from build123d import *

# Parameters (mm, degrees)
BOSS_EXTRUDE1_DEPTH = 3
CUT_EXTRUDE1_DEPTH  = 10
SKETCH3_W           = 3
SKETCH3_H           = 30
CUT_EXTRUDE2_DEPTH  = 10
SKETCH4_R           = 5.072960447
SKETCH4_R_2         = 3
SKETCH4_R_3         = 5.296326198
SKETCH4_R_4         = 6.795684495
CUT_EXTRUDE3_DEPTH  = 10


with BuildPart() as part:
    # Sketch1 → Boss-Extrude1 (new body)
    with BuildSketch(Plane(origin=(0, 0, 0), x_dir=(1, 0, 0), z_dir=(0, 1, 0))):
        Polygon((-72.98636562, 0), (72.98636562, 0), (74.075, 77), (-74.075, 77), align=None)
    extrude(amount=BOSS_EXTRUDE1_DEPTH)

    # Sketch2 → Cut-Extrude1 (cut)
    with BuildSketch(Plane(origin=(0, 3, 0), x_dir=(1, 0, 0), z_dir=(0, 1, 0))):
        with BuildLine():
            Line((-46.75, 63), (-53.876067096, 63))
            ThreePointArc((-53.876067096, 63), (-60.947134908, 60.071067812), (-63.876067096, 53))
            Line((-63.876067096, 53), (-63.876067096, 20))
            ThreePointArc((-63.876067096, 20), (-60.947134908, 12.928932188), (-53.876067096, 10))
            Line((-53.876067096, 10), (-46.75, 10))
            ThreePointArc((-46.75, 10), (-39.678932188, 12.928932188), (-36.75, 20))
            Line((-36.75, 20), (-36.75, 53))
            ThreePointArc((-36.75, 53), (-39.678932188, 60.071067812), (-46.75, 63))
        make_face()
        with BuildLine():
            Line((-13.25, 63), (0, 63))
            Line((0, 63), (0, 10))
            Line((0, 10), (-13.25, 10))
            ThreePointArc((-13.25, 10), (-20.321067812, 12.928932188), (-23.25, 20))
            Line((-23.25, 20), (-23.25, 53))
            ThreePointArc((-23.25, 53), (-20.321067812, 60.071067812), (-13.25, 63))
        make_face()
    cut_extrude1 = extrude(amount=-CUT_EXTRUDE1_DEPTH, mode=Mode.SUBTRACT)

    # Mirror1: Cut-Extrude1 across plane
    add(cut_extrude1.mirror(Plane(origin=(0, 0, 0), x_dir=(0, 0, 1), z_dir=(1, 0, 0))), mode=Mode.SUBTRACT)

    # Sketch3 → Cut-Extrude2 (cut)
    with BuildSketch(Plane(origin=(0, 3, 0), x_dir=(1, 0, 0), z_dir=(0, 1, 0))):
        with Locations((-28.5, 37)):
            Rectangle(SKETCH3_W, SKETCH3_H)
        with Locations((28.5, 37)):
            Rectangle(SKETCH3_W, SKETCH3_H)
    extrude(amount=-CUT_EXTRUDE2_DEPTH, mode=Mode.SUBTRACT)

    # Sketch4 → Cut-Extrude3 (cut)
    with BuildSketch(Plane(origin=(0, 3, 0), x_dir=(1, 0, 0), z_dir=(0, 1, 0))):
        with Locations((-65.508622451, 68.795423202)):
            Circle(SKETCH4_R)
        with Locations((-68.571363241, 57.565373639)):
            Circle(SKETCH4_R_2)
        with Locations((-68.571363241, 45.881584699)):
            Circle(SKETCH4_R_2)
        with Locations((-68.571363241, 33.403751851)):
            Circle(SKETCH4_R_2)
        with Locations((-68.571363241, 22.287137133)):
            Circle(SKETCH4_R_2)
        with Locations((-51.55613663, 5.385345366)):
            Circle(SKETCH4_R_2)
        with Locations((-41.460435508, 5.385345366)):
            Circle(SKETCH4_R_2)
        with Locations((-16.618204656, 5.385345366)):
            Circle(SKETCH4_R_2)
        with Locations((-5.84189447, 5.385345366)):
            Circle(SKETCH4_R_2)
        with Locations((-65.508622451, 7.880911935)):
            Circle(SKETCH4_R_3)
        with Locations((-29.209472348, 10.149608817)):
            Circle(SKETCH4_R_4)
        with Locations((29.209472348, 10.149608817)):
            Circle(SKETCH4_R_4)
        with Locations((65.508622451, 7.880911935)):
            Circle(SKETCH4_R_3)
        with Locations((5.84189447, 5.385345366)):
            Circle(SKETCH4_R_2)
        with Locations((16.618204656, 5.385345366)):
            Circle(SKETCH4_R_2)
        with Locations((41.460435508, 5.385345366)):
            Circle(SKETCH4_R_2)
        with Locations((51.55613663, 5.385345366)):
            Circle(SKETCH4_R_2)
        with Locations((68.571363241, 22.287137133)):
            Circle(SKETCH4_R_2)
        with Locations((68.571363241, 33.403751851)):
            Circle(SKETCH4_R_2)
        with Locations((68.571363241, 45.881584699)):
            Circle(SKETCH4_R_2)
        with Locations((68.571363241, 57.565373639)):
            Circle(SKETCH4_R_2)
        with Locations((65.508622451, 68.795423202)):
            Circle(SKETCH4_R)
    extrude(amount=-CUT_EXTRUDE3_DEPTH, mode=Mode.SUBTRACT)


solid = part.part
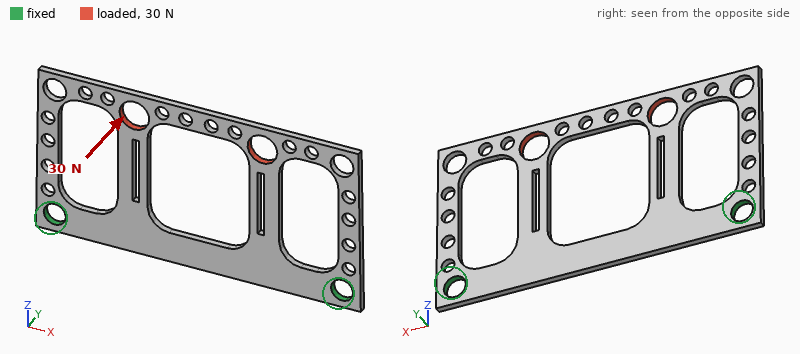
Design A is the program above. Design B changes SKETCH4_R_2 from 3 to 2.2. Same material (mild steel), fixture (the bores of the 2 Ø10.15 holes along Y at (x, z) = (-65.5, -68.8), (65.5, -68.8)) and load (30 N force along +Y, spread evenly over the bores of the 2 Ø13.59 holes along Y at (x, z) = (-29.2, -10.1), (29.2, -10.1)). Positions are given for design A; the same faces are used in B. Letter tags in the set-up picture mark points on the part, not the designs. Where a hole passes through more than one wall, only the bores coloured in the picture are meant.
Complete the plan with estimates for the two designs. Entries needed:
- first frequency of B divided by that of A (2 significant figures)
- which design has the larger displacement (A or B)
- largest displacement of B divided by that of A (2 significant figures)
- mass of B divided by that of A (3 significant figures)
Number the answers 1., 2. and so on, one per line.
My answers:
1. 1.0
2. A
3. 0.90
4. 1.04
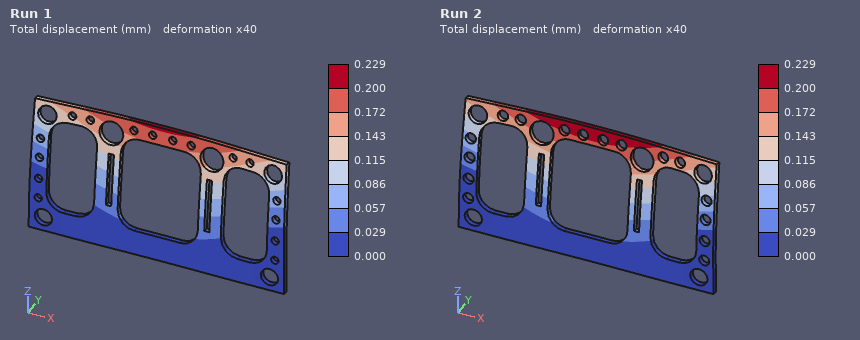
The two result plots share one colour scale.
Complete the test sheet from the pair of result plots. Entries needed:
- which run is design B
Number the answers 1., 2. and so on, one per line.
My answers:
1. Run 1
